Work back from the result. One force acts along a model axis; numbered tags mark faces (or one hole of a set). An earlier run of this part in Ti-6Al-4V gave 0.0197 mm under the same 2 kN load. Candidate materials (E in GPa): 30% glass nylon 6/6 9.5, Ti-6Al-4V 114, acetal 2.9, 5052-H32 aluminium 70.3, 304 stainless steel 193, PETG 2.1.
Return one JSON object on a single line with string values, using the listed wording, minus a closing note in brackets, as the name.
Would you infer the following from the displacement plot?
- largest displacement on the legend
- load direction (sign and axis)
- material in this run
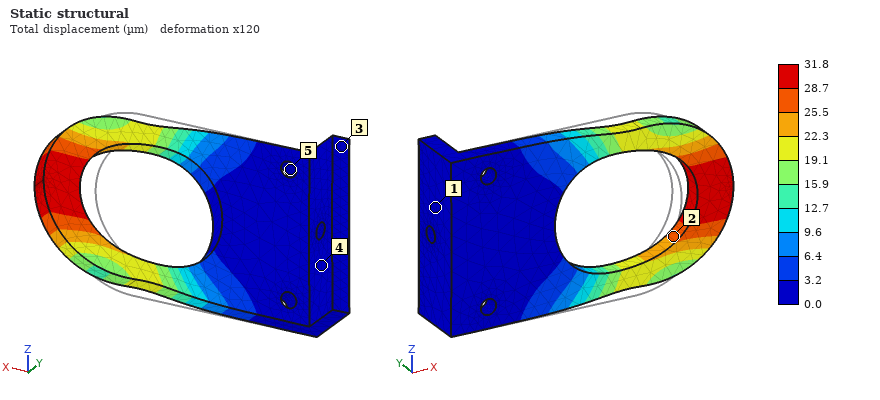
{"largest displacement on the legend": "31.8 µm", "load direction": "+X", "material in this run": "5052-H32 aluminium"}
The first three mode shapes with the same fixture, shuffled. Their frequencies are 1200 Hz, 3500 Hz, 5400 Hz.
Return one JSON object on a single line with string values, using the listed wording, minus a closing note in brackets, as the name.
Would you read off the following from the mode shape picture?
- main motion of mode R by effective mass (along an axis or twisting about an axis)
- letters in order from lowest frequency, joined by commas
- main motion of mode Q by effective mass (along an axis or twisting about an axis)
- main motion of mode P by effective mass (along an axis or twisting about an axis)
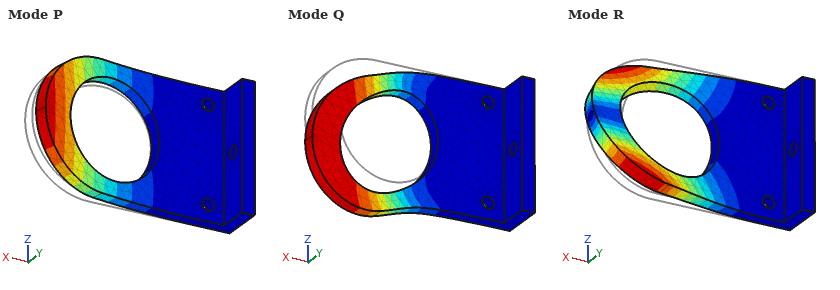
{"main motion of mode R by effective mass": "twisting about X", "letters in order from lowest frequency, joined by commas": "P, R, Q", "main motion of mode Q by effective mass": "along Z", "main motion of mode P by effective mass": "along Y"}
